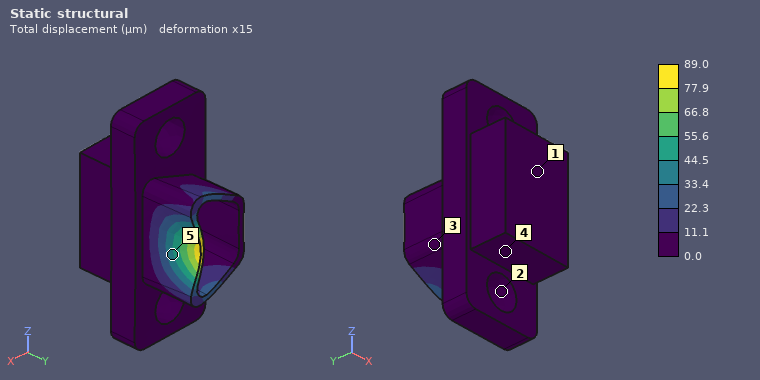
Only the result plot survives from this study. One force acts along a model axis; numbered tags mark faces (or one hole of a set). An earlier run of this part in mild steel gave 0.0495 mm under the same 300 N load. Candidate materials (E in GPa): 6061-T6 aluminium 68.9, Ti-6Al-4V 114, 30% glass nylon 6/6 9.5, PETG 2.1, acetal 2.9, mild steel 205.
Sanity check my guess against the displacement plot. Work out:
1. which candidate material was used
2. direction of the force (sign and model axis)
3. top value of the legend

Ti-6Al-4V
-X
89.0 µm
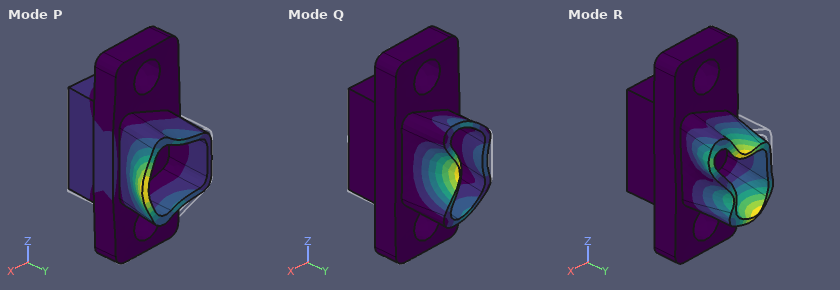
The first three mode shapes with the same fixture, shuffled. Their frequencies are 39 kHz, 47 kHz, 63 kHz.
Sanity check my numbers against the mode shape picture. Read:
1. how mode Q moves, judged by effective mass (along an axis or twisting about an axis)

along X
